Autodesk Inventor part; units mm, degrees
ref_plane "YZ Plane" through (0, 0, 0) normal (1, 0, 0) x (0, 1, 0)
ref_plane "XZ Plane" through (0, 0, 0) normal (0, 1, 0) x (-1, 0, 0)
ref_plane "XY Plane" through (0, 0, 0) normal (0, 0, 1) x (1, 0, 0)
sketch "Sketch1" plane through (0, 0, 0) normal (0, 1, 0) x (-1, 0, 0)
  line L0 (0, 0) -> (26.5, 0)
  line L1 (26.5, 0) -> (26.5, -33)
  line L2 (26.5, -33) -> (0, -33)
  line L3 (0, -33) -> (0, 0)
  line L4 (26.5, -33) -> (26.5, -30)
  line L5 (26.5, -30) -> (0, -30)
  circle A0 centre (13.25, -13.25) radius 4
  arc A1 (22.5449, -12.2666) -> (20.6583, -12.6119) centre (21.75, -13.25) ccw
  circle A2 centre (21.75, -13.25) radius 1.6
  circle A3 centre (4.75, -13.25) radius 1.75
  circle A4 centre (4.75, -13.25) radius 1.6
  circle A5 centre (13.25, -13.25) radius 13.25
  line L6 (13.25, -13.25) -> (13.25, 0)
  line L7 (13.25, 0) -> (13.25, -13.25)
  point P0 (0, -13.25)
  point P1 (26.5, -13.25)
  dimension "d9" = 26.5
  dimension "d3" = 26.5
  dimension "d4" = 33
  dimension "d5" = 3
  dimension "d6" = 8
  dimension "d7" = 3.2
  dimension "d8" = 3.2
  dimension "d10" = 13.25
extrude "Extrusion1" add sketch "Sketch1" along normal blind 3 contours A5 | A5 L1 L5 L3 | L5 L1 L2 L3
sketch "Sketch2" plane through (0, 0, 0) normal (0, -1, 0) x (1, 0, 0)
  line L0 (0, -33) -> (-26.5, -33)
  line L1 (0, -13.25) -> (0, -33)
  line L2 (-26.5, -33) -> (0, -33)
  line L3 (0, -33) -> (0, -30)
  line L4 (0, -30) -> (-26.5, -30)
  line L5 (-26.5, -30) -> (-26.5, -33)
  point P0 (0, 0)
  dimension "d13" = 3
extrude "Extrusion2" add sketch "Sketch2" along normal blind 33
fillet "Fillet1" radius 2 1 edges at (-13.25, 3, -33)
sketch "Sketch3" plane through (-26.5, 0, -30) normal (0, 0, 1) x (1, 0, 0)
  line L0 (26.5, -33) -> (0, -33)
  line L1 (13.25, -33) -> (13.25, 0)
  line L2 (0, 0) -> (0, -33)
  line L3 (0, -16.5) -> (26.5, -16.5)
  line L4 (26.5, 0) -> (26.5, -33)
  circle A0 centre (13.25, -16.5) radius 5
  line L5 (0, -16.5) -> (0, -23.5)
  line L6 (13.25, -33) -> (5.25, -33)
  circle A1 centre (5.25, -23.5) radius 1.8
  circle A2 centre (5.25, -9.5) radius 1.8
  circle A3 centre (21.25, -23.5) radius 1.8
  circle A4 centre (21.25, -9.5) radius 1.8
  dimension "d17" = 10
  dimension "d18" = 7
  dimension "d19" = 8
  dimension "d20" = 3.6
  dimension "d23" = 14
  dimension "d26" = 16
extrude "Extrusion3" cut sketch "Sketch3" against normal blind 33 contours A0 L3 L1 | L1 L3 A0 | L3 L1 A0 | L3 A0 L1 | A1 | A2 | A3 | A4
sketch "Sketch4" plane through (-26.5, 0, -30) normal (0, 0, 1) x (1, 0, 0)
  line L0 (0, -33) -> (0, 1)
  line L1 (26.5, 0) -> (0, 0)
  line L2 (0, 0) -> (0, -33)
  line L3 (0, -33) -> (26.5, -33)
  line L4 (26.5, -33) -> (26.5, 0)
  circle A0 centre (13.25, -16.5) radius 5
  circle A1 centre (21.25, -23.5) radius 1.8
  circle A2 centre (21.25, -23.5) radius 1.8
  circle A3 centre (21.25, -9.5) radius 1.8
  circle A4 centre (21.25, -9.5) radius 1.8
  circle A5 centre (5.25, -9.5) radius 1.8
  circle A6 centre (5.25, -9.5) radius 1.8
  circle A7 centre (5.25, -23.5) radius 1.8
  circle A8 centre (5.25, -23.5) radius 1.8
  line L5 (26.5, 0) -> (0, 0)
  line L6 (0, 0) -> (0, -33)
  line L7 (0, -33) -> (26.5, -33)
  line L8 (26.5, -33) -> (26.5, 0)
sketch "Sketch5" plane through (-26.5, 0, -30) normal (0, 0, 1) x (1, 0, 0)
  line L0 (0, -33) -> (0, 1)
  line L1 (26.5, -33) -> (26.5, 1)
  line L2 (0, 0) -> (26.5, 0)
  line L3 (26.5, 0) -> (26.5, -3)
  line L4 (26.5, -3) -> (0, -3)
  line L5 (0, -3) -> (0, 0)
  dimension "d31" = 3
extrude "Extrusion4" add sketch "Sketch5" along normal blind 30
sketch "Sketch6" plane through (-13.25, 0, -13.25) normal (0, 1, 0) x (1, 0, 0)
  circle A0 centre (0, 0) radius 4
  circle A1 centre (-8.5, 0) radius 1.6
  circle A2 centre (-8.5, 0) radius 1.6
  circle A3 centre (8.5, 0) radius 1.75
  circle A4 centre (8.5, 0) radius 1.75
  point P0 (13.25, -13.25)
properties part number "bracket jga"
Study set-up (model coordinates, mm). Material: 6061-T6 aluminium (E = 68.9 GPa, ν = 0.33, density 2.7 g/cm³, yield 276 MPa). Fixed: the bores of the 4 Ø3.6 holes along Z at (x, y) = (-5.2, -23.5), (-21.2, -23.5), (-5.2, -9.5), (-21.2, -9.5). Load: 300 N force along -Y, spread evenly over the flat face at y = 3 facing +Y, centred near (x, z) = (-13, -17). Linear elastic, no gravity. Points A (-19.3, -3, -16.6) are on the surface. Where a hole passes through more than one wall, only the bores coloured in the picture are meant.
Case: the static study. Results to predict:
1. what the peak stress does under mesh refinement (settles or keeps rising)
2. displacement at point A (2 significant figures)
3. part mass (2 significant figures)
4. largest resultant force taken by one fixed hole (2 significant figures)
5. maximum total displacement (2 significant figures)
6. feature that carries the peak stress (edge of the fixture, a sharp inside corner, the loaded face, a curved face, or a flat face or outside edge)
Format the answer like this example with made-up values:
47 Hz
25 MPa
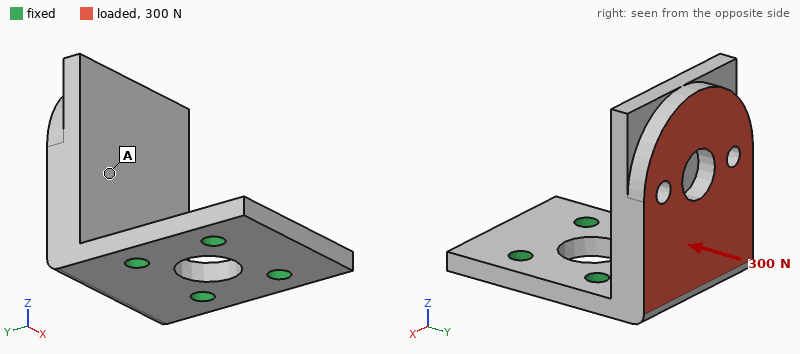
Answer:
keeps rising
0.12 mm
18 g
150 N
0.27 mm
edge of the fixture
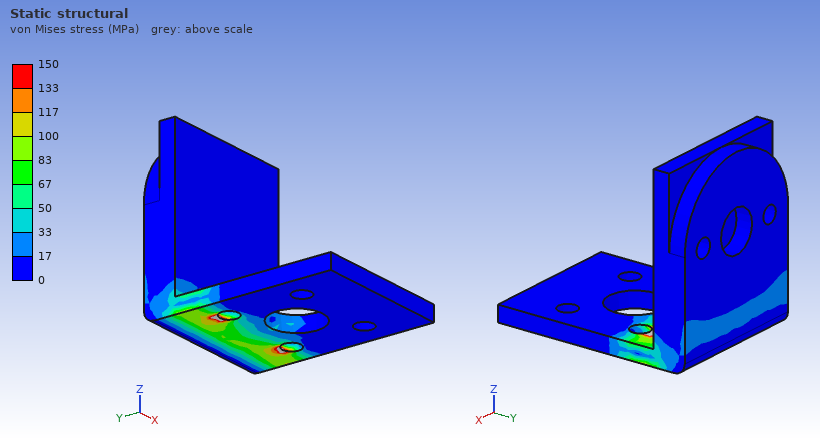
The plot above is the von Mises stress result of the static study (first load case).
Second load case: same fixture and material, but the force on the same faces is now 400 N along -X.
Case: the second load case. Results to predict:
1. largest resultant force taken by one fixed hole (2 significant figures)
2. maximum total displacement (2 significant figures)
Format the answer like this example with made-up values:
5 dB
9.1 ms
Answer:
450 N
44 µm
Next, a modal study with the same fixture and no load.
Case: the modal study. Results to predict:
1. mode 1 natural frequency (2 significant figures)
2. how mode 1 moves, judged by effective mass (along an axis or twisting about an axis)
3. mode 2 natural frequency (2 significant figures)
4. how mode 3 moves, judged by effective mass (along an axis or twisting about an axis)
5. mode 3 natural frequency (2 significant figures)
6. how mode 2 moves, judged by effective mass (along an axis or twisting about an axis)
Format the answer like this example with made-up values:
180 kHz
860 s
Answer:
1800 Hz
along Y
4800 Hz
along Z
11 kHz
along X
